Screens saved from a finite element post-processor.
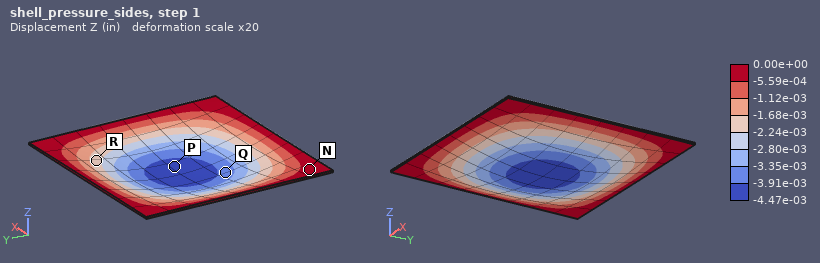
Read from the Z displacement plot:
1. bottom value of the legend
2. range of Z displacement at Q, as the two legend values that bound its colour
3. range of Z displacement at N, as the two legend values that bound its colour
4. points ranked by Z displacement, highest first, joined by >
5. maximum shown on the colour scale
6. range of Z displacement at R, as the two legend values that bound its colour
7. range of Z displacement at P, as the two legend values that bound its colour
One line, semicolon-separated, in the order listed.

-4.47e-03 in; -3.91e-03 to -3.35e-03 in; -5.59e-04 to 0.00e+00 in; N > R > Q > P; 0.00e+00 in; -2.24e-03 to -1.68e-03 in; -4.47e-03 to -3.91e-03 in
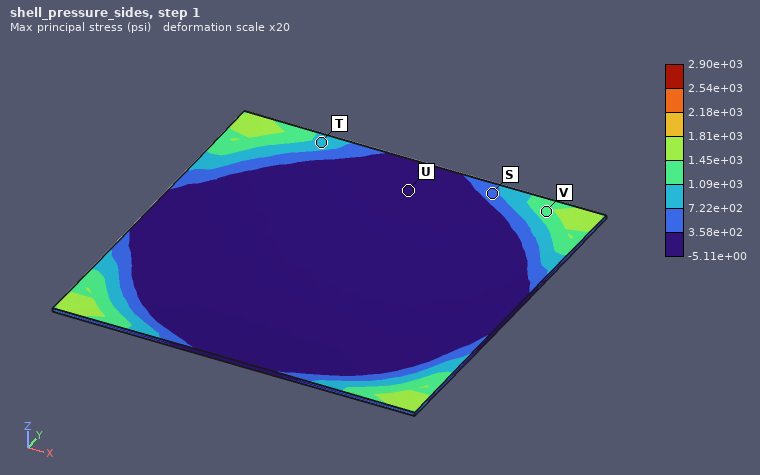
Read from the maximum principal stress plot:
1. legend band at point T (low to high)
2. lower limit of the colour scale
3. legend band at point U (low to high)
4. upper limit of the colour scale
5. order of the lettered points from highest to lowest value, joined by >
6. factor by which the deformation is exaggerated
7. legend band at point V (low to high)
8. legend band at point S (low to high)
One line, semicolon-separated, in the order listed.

7.22e+02 to 1.09e+03 psi; -5.11e+00 psi; -5.11e+00 to 3.58e+02 psi; 2.90e+03 psi; V > T > S > U; 20; 1.09e+03 to 1.45e+03 psi; 3.58e+02 to 7.22e+02 psi
